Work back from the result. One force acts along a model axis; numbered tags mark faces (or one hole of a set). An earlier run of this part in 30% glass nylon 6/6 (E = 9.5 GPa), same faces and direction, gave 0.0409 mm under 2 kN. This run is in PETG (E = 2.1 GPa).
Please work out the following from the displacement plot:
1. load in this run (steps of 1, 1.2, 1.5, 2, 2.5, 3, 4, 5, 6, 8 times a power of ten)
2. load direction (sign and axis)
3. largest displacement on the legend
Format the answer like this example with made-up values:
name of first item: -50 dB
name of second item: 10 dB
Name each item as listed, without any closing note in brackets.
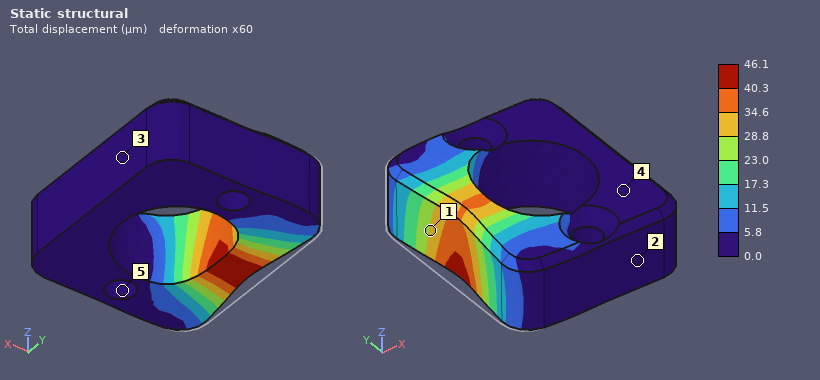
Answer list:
load in this run: 500 N
load direction: +X
largest displacement on the legend: 46.1 µm
